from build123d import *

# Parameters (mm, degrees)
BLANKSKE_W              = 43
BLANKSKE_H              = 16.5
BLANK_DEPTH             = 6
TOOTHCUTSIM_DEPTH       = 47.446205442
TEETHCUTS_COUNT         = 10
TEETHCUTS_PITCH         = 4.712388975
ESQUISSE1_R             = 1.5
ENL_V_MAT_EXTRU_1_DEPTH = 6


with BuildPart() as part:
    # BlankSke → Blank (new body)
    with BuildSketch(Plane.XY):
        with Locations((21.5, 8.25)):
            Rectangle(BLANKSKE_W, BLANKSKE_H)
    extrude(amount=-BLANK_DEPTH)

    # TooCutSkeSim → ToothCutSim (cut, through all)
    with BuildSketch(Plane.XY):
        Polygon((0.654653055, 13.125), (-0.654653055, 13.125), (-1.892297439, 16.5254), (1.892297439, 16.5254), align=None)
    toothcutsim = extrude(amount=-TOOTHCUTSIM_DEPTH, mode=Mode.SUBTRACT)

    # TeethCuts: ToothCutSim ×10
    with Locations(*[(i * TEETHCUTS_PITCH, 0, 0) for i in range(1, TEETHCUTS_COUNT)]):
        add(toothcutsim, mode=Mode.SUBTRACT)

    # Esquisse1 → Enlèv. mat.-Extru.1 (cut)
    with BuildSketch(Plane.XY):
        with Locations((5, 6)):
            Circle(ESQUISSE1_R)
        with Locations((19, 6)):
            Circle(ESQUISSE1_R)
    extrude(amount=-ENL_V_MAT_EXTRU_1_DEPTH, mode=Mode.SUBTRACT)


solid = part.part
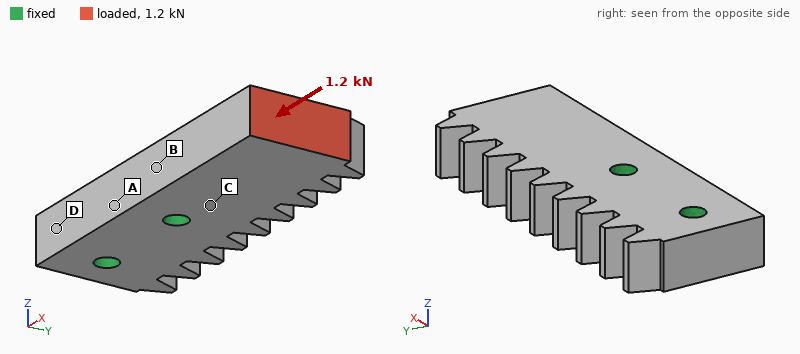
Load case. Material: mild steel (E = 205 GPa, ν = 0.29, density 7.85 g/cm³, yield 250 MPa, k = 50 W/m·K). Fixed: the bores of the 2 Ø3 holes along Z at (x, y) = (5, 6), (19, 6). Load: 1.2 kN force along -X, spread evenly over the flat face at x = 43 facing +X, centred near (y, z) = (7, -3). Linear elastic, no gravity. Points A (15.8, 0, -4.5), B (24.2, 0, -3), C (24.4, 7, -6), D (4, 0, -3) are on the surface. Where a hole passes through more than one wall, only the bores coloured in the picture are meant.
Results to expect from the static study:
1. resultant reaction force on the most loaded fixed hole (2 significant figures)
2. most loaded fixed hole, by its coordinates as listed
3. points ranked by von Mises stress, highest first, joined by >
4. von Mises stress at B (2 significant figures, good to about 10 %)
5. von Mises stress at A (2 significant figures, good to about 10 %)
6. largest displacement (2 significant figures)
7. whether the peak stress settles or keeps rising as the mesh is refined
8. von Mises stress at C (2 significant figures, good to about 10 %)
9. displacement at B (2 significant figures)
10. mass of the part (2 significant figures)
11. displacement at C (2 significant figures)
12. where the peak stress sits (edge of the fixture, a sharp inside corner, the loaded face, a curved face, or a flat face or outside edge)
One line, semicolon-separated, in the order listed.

1.0 kN; (19, 6); C > B > A > D; 11 MPa; 6.1 MPa; 2.0 µm; keeps rising; 20 MPa; 0.49 µm; 29 g; 0.50 µm; edge of the fixture
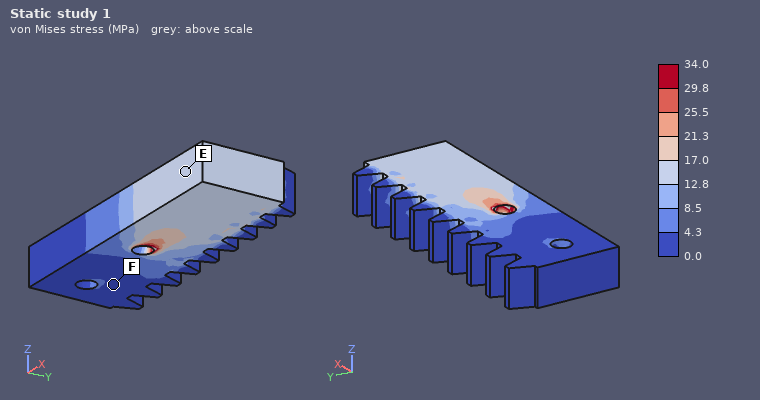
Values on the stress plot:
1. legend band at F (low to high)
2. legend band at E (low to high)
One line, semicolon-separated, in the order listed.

0.0 to 4.3 MPa; 12.8 to 17.0 MPa
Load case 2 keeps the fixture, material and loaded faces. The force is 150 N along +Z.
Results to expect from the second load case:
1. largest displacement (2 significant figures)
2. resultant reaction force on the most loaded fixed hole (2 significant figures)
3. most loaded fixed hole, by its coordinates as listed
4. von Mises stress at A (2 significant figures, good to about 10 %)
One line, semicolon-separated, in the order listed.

15 µm; 220 N; (19, 6); 8.2 MPa
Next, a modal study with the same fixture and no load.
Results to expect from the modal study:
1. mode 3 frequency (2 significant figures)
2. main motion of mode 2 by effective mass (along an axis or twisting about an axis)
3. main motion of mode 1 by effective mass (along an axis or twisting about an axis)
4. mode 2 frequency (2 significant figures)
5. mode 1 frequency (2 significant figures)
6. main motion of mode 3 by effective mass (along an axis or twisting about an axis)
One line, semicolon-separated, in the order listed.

20 kHz; along Y; along Z; 12 kHz; 7700 Hz; twisting about X
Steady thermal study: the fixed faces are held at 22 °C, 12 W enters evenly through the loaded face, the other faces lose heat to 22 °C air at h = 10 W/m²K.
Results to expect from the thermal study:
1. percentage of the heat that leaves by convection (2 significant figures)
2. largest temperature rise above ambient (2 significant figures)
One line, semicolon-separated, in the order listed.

3.5 %; 71 K
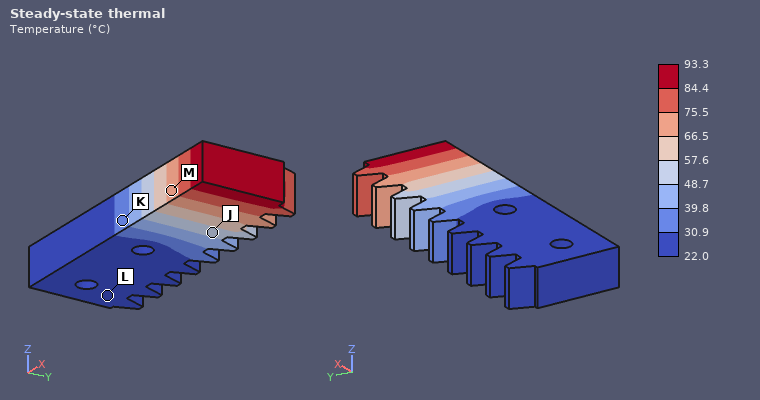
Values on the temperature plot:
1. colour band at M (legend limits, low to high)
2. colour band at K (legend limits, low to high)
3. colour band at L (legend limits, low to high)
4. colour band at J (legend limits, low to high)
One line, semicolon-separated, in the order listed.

66.5 to 75.5 °C; 30.9 to 39.8 °C; 22.0 to 30.9 °C; 48.7 to 57.6 °C
